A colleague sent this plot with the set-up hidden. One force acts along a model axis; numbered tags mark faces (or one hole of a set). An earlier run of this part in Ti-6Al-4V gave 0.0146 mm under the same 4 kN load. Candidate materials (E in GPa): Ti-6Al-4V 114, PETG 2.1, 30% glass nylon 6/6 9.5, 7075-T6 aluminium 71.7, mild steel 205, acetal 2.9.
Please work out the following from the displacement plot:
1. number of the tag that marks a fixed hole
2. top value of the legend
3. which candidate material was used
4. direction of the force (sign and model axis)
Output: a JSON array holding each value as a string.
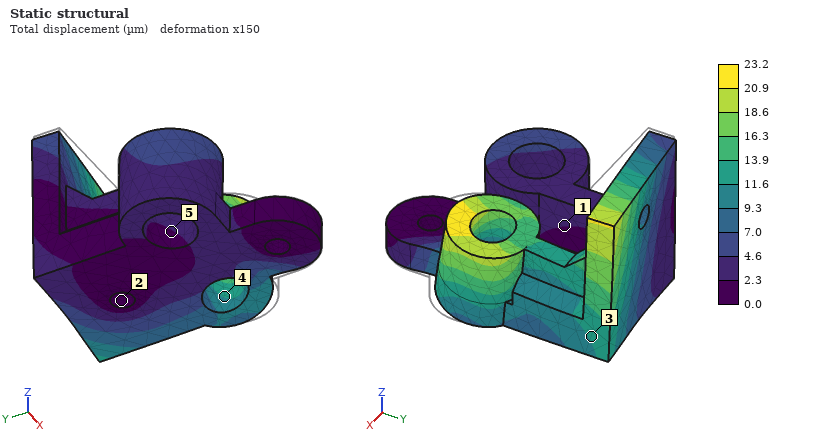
["2", "23.2 µm", "7075-T6 aluminium", "+Y"]
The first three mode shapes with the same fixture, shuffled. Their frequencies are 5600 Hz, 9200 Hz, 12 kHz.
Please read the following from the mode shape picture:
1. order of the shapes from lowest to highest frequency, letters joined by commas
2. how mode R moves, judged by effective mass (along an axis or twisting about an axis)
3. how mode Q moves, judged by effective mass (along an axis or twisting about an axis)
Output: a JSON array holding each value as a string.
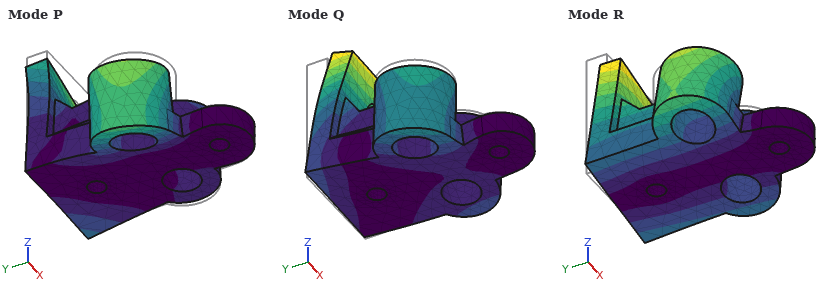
["R, Q, P", "along X", "along Y"]
